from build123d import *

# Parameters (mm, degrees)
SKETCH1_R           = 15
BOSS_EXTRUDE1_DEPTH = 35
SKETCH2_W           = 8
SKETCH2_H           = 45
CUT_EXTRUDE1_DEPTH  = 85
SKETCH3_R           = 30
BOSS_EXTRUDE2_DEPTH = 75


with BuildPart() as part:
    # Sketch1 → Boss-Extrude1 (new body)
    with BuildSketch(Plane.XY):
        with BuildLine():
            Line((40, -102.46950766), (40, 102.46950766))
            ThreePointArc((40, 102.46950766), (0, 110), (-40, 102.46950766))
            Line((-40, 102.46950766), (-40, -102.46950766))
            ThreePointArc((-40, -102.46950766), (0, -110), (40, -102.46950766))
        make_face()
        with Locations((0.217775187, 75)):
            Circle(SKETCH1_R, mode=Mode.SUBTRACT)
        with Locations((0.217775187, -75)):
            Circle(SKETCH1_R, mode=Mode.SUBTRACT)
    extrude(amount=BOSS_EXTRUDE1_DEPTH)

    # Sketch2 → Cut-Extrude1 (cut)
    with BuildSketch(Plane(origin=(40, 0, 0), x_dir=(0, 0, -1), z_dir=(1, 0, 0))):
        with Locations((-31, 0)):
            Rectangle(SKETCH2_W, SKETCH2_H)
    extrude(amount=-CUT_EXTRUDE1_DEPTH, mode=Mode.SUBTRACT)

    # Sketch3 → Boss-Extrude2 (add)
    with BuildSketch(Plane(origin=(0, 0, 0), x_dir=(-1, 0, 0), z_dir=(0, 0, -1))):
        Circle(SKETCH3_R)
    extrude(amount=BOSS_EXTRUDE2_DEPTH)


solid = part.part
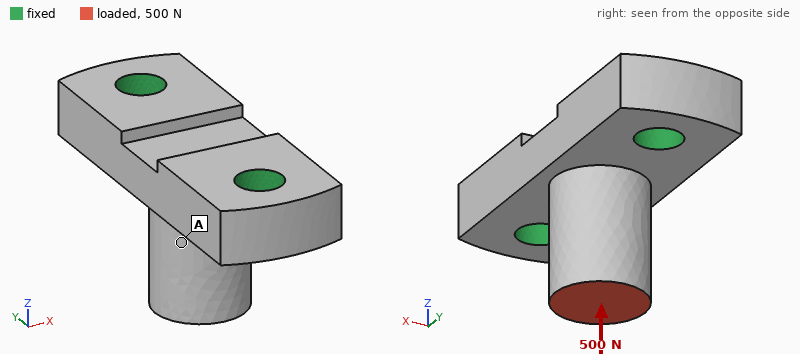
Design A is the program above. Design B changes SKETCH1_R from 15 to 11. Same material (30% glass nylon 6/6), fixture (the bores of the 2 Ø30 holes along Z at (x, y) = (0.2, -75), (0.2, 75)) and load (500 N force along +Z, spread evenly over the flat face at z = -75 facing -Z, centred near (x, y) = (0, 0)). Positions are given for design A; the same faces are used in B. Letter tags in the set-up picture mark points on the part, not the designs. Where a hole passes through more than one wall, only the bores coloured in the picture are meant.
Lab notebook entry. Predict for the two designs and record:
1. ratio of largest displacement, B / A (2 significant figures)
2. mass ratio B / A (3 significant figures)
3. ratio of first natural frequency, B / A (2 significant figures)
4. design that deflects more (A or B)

1.2
1.03
0.93
B
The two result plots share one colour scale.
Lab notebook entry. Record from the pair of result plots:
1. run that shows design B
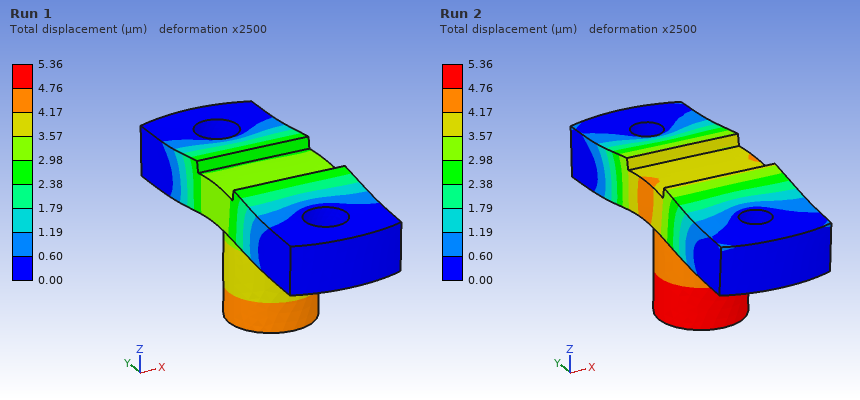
Run 2
